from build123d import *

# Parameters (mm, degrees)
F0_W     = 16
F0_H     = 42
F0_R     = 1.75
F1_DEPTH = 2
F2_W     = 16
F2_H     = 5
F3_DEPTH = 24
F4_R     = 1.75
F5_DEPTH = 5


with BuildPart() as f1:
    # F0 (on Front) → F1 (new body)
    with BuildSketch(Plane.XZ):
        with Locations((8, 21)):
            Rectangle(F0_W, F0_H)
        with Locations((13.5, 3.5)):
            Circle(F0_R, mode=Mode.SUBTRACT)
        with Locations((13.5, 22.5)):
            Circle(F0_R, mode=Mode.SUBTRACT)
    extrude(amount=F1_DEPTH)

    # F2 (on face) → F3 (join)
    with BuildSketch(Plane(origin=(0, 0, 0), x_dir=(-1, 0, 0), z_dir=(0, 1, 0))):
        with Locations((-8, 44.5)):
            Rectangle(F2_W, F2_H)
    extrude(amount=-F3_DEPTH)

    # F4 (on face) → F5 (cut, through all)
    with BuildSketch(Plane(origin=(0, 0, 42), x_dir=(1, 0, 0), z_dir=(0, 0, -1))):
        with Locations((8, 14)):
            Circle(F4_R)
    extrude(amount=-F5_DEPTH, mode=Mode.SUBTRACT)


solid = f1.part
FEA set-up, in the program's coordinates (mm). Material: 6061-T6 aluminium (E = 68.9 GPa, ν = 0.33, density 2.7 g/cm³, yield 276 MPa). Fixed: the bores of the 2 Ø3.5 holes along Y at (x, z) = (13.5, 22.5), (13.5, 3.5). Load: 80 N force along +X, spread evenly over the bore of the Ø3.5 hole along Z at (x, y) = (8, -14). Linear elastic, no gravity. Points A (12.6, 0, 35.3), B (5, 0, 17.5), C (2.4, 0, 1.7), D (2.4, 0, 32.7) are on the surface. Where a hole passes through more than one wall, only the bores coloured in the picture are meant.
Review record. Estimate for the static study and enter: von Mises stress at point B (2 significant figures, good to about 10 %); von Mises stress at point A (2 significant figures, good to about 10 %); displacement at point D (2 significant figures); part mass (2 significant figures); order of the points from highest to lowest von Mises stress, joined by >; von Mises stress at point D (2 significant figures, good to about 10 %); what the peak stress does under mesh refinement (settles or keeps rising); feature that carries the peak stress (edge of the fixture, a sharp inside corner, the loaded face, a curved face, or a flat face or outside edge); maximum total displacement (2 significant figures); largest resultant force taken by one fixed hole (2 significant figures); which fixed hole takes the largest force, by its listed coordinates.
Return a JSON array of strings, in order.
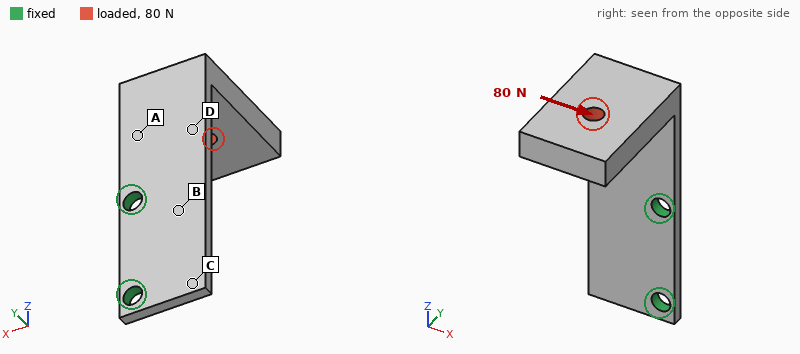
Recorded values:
["43 MPa", "81 MPa", "0.10 mm", "8.6 g", "A > D > B > C", "63 MPa", "keeps rising", "edge of the fixture", "0.48 mm", "170 N", "(13.5, 22.5)"]
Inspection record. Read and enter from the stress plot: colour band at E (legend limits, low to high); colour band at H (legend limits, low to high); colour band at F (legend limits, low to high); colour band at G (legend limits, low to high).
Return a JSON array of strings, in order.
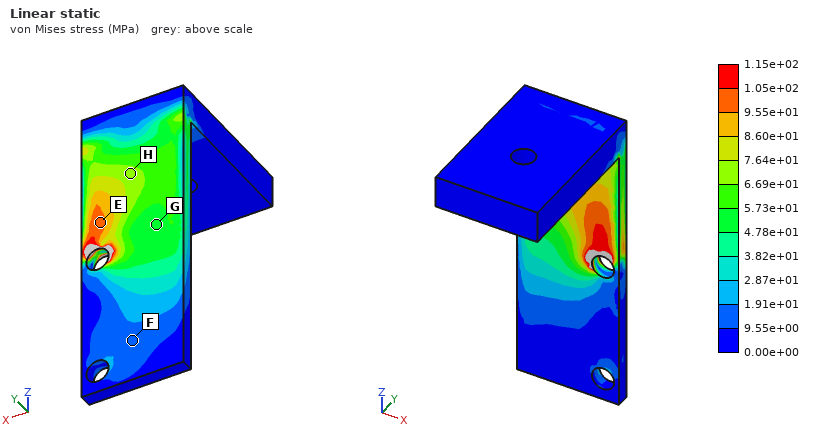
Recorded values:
["9.55e+01 to 1.05e+02 MPa", "6.69e+01 to 7.64e+01 MPa", "9.55e+00 to 1.91e+01 MPa", "4.78e+01 to 5.73e+01 MPa"]
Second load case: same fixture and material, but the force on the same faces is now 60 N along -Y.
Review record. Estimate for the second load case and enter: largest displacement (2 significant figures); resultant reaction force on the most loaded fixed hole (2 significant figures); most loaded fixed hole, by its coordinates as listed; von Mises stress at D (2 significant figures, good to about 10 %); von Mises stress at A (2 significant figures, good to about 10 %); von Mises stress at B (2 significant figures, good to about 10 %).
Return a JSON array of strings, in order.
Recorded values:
["0.60 mm", "80 N", "(13.5, 22.5)", "61 MPa", "52 MPa", "28 MPa"]
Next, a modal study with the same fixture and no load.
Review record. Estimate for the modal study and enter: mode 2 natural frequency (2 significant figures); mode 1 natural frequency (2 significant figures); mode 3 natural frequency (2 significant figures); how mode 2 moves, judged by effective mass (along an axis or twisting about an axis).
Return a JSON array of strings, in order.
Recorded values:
["1200 Hz", "720 Hz", "2800 Hz", "along X"]
